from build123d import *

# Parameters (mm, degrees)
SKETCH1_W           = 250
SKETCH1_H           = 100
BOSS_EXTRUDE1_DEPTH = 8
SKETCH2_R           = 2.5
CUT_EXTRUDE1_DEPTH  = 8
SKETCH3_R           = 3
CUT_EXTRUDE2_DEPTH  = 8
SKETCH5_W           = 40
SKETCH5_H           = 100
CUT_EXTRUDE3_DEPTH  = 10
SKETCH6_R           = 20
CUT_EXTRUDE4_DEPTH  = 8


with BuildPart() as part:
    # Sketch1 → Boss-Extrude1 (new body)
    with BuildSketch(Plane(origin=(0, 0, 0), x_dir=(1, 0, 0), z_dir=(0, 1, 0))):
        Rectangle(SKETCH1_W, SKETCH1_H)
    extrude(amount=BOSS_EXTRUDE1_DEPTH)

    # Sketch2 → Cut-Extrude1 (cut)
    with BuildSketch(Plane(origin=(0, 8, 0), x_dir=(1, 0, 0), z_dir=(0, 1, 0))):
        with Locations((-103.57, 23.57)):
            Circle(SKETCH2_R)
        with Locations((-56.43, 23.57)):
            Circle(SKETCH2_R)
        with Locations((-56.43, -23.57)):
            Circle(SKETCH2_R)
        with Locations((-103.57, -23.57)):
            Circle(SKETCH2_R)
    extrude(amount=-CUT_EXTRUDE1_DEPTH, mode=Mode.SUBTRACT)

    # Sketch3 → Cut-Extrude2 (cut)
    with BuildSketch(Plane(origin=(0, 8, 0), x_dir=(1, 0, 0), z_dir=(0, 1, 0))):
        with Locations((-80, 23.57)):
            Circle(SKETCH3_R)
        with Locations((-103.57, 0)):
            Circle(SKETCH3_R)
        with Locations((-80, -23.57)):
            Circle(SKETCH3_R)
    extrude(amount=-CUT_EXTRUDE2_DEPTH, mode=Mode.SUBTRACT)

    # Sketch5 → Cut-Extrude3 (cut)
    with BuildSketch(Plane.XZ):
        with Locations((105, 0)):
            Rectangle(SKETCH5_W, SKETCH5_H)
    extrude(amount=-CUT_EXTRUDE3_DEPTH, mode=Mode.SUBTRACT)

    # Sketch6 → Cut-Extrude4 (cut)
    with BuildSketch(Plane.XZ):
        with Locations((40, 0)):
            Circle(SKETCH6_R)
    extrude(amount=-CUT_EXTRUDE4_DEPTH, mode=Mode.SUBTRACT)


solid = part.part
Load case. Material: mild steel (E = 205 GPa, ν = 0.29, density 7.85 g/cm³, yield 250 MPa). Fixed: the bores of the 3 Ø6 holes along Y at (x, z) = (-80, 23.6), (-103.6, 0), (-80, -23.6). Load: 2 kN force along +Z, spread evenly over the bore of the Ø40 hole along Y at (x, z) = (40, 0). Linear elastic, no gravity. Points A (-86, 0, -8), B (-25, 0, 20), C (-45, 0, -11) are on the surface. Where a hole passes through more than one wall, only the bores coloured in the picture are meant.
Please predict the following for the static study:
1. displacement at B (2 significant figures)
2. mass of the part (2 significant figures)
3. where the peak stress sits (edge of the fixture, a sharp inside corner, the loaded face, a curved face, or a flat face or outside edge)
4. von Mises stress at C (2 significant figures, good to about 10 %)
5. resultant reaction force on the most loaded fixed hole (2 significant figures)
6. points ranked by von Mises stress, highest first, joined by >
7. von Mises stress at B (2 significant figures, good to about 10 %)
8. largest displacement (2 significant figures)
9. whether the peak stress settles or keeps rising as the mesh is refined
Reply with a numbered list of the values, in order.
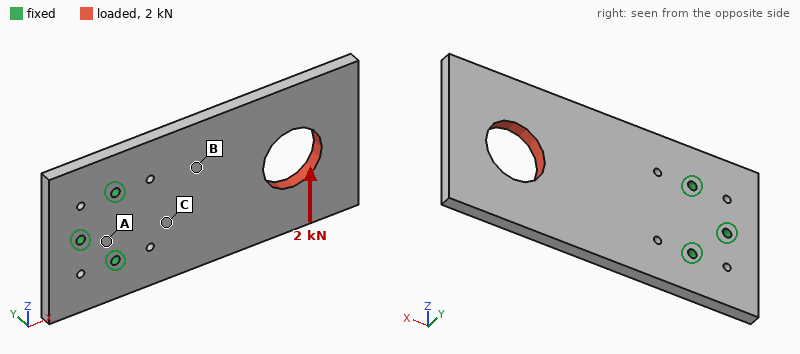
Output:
1. 7.9 µm
2. 1.2 kg
3. edge of the fixture
4. 8.8 MPa
5. 4.4 kN
6. C > B > A
7. 6.6 MPa
8. 30 µm
9. keeps rising
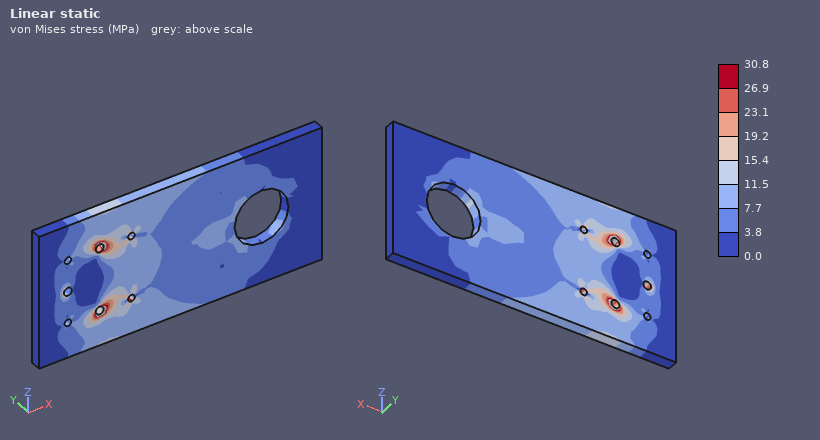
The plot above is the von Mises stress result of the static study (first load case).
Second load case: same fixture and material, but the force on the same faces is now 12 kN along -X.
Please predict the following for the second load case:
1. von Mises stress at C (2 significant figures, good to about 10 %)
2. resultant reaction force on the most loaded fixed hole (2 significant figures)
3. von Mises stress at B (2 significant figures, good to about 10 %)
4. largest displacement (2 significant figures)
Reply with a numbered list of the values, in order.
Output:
1. 17 MPa
2. 5.1 kN
3. 15 MPa
4. 16 µm
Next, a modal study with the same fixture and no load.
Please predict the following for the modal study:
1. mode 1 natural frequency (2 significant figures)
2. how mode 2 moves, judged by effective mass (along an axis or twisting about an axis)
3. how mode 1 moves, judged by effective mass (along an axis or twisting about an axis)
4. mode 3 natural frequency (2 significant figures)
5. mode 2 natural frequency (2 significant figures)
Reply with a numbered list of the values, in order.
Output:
1. 250 Hz
2. twisting about X
3. along Y
4. 1400 Hz
5. 820 Hz
